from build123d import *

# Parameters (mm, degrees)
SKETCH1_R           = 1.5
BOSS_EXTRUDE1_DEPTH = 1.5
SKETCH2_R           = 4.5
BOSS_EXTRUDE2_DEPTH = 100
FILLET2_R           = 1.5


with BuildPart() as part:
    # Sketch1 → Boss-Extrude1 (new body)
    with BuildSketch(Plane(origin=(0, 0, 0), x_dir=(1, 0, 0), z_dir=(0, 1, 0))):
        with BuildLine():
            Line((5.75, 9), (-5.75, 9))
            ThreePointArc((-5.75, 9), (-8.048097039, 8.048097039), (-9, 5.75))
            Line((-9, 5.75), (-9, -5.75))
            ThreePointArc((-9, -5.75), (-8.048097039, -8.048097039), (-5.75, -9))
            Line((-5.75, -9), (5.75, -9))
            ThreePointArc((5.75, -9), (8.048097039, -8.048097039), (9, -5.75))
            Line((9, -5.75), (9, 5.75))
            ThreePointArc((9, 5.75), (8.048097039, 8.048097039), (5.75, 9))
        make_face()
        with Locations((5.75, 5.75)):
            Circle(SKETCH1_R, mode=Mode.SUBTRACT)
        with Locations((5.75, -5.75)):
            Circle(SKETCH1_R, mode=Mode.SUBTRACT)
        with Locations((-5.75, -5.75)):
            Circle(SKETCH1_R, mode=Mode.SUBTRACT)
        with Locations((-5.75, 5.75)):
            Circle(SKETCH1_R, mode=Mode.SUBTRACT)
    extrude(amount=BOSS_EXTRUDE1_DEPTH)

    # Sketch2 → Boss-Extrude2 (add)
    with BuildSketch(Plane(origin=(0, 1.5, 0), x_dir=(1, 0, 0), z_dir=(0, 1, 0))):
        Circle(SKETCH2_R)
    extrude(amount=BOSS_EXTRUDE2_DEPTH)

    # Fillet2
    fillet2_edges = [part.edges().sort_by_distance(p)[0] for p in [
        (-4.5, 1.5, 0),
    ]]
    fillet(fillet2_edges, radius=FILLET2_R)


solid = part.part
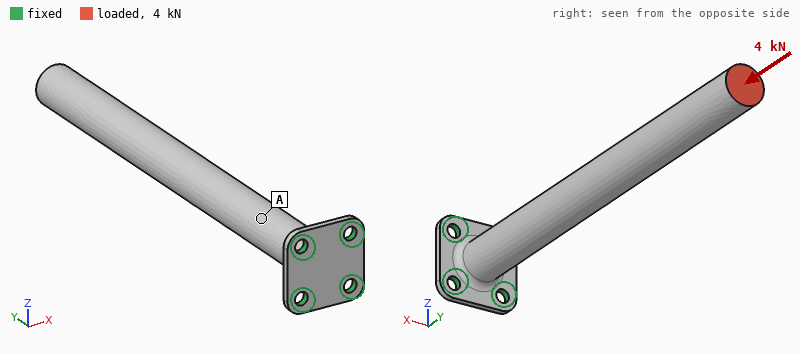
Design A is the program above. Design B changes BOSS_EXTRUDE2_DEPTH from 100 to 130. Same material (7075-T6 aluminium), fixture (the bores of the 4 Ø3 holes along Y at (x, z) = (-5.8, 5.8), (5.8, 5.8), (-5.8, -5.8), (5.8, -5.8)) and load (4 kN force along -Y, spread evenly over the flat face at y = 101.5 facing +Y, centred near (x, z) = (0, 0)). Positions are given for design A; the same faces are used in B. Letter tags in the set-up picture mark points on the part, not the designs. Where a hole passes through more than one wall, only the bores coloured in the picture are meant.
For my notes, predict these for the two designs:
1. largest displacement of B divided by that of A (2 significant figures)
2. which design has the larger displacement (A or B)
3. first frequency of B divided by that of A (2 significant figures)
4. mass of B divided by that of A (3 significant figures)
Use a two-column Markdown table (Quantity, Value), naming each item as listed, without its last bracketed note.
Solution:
| Quantity | Value |
|---|---|
| largest displacement of B divided by that of A | 1.2 |
| which design has the larger displacement | B |
| first frequency of B divided by that of A | 0.61 |
| mass of B divided by that of A | 1.28 |
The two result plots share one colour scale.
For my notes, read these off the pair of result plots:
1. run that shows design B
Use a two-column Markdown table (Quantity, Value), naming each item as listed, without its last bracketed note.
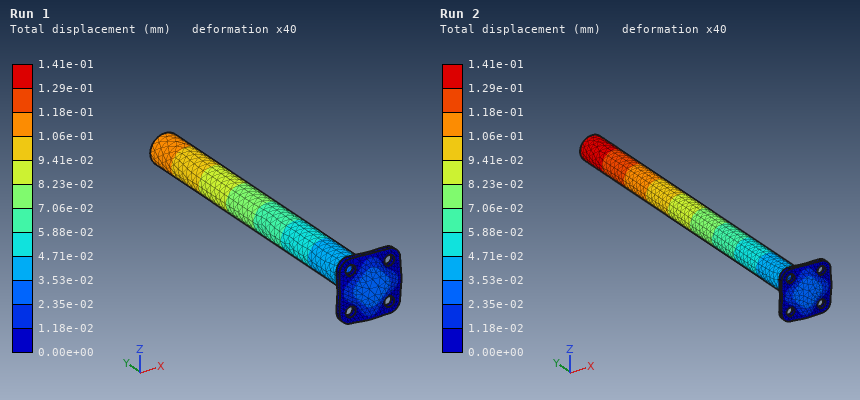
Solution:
| Quantity | Value |
|---|---|
| run that shows design B | Run 2 |
